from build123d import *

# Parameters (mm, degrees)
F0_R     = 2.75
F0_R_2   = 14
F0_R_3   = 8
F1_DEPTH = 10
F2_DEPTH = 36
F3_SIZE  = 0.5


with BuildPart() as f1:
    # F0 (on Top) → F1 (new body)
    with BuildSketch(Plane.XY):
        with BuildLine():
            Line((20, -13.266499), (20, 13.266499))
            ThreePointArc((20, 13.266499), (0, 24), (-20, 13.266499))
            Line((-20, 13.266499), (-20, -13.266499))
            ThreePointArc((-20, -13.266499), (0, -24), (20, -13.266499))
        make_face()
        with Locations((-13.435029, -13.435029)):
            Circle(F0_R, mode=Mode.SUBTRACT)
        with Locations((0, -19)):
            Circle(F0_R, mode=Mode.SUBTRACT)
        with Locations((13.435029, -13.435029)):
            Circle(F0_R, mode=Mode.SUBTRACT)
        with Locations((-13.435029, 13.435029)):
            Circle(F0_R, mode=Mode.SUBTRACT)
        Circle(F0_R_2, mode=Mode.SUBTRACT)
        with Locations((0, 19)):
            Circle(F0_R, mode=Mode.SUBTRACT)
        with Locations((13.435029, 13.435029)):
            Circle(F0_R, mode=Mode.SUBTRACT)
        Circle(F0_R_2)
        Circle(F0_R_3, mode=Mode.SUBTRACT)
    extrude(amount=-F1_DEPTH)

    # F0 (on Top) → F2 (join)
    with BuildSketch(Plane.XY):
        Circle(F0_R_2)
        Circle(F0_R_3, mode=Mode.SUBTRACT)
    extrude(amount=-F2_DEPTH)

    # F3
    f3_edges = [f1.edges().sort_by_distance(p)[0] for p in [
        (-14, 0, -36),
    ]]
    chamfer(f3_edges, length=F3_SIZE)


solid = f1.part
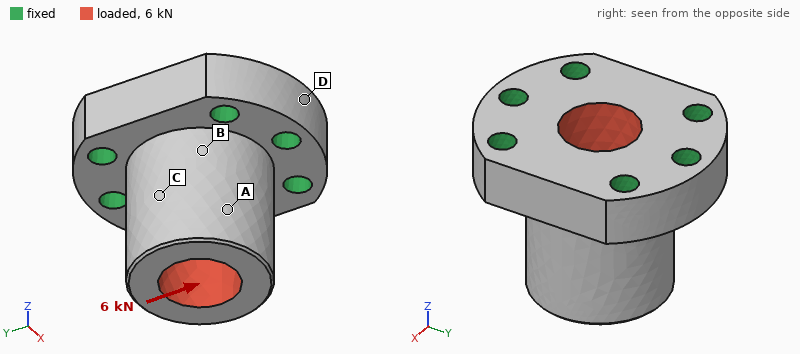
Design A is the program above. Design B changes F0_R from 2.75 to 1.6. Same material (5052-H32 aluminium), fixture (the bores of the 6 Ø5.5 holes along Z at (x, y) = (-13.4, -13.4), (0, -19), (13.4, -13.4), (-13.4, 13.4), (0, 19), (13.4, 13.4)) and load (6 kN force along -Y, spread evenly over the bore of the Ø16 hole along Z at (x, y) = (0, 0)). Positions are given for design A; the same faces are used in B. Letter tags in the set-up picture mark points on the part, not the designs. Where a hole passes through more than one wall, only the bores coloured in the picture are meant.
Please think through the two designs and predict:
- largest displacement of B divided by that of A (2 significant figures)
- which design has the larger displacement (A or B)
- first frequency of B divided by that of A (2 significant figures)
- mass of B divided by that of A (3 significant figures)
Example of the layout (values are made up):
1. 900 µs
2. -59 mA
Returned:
1. 1.1
2. B
3. 0.94
4. 1.04
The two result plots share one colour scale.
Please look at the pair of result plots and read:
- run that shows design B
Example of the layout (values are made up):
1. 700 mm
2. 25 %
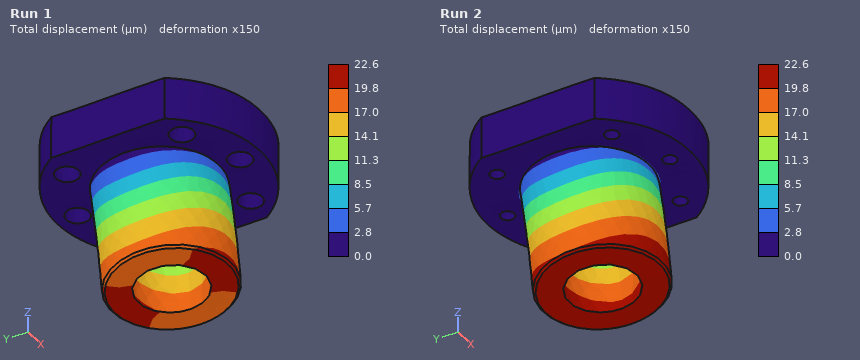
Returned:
1. Run 2
